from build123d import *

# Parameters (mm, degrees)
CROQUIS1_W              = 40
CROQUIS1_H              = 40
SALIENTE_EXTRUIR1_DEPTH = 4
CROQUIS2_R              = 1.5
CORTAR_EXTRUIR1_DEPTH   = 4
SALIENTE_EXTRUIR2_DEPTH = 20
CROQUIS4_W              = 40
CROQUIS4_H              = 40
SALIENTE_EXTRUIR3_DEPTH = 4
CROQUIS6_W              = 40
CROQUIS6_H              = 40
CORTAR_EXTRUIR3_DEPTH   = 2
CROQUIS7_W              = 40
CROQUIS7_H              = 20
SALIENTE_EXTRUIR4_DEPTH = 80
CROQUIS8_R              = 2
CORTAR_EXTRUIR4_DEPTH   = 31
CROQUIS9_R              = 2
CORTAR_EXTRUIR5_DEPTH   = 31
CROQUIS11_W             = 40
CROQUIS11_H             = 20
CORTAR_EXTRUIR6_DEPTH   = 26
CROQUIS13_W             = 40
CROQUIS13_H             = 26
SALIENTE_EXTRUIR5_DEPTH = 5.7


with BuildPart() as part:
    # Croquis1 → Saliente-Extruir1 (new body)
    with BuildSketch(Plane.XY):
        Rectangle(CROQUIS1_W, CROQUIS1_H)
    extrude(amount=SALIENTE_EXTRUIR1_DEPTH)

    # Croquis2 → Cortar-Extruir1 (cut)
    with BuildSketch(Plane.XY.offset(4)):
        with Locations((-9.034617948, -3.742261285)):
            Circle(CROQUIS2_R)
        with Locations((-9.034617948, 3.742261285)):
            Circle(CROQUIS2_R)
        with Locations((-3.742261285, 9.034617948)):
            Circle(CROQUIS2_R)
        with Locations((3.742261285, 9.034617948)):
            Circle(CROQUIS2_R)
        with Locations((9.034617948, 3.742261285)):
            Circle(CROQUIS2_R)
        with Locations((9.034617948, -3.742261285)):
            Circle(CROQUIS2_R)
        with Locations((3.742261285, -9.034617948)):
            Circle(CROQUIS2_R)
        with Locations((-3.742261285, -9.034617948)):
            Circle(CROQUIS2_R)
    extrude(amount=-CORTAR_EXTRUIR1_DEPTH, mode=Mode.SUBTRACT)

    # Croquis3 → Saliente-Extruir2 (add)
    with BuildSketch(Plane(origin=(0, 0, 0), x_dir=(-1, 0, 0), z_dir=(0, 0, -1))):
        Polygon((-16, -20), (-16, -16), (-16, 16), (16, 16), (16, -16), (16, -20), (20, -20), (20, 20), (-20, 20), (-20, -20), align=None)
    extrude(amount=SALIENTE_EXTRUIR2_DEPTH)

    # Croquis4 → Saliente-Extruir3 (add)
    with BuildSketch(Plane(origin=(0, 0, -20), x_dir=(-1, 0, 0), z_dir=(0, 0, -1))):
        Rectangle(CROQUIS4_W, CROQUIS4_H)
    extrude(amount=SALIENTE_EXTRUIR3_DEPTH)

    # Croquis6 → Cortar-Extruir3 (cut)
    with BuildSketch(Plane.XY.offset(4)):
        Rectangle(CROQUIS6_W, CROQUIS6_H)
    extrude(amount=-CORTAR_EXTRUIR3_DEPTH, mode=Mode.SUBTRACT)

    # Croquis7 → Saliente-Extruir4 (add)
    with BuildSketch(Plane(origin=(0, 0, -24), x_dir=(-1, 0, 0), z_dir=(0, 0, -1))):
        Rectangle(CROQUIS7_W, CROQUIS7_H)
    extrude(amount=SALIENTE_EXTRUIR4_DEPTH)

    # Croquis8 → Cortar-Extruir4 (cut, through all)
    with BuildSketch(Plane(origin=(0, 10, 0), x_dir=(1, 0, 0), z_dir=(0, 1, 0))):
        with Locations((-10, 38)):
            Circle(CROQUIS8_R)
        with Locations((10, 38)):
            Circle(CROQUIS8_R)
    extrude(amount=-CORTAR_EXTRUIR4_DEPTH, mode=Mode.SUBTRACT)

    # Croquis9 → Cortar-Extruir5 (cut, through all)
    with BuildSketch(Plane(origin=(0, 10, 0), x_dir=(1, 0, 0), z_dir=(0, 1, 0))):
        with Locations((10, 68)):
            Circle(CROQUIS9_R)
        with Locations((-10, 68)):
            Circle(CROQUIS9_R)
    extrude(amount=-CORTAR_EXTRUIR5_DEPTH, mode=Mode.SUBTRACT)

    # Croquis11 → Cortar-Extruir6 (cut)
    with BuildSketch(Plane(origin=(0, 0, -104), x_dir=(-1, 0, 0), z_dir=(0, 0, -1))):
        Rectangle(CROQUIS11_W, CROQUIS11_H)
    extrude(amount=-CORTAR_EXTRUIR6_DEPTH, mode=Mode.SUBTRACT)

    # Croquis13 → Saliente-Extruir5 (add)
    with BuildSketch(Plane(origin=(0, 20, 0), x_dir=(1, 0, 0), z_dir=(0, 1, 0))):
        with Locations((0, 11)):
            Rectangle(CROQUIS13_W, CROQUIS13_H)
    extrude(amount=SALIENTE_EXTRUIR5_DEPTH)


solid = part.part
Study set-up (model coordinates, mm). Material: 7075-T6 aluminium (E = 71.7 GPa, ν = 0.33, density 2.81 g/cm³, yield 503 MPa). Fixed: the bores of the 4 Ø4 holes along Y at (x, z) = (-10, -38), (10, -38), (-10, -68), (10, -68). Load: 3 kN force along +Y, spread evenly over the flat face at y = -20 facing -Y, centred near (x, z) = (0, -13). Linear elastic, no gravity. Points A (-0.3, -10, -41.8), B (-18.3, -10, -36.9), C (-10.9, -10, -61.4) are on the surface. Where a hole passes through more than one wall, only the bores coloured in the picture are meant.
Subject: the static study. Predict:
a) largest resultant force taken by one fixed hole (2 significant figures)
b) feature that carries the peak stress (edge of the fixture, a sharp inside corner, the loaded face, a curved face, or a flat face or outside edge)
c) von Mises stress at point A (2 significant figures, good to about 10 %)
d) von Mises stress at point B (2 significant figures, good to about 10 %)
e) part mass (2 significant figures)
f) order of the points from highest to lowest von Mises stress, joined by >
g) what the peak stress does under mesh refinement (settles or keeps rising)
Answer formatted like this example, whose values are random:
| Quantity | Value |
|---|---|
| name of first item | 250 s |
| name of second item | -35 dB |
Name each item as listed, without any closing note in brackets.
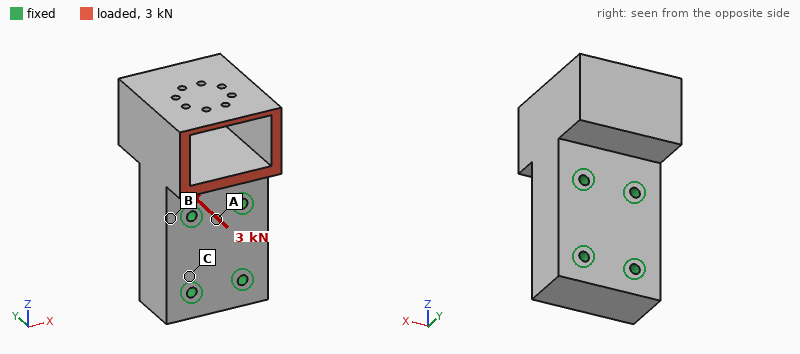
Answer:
| Quantity | Value |
|---|---|
| largest resultant force taken by one fixed hole | 1.8 kN |
| feature that carries the peak stress | edge of the fixture |
| von Mises stress at point A | 11 MPa |
| von Mises stress at point B | 19 MPa |
| part mass | 190 g |
| order of the points from highest to lowest von Mises stress, joined by > | B > A > C |
| what the peak stress does under mesh refinement | keeps rising |
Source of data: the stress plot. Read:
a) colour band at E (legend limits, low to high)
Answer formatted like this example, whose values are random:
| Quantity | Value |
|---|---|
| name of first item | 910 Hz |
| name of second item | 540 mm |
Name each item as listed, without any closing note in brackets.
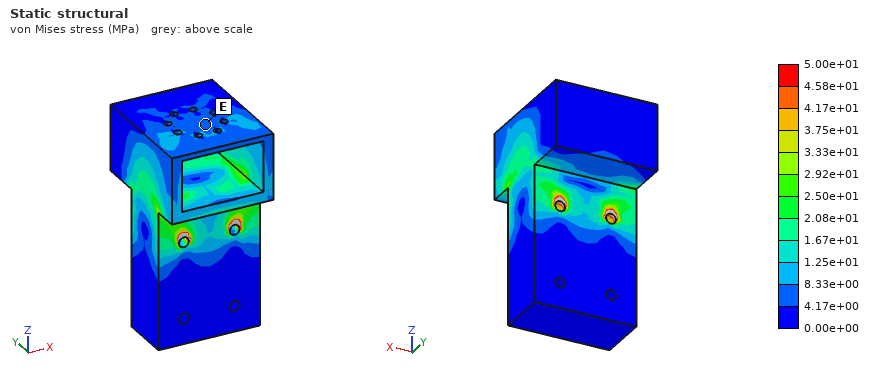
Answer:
| Quantity | Value |
|---|---|
| colour band at E | 4.17e+00 to 8.33e+00 MPa |
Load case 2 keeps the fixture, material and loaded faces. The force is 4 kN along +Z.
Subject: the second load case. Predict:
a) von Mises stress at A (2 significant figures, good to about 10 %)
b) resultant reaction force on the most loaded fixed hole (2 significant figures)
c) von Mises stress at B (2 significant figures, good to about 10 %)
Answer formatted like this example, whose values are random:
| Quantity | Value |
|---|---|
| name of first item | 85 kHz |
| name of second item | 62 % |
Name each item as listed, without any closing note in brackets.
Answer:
| Quantity | Value |
|---|---|
| von Mises stress at A | 11 MPa |
| resultant reaction force on the most loaded fixed hole | 1.8 kN |
| von Mises stress at B | 27 MPa |
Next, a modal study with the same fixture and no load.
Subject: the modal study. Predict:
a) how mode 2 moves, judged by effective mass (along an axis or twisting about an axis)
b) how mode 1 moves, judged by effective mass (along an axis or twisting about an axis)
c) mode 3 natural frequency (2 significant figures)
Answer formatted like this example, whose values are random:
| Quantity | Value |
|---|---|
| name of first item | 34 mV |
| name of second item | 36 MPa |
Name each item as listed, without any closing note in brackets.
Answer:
| Quantity | Value |
|---|---|
| how mode 2 moves, judged by effective mass | along X |
| how mode 1 moves, judged by effective mass | along Y |
| mode 3 natural frequency | 8700 Hz |
